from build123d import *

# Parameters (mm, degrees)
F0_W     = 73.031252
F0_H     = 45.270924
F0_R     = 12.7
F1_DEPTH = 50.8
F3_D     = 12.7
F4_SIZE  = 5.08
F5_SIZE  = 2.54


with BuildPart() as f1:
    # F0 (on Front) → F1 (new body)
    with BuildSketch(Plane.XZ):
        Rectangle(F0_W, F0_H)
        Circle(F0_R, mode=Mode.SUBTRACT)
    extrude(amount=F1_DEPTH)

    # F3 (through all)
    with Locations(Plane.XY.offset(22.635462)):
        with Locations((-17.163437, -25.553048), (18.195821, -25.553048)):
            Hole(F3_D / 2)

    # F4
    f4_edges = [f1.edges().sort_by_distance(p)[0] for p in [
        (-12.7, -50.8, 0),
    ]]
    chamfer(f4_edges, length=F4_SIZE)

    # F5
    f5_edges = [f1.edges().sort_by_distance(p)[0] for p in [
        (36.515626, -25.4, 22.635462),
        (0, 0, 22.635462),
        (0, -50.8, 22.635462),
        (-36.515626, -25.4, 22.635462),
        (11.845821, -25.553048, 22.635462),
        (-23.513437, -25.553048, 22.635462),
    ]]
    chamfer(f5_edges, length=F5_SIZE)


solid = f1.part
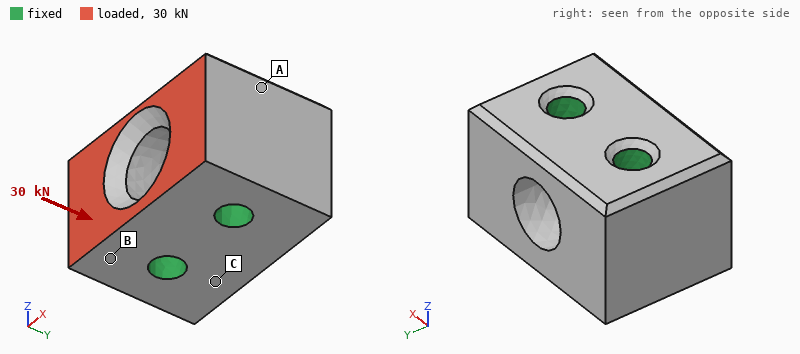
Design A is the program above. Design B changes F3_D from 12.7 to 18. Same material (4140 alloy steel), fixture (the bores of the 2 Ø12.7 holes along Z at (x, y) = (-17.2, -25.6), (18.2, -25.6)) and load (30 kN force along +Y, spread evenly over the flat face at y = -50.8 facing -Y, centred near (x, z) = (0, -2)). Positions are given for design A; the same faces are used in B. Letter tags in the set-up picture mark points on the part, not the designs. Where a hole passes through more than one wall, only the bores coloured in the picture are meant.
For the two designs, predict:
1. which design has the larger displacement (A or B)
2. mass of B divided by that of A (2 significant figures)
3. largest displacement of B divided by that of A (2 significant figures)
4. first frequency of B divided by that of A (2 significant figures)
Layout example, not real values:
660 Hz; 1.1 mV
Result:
A; 0.92; 0.83; 1.3
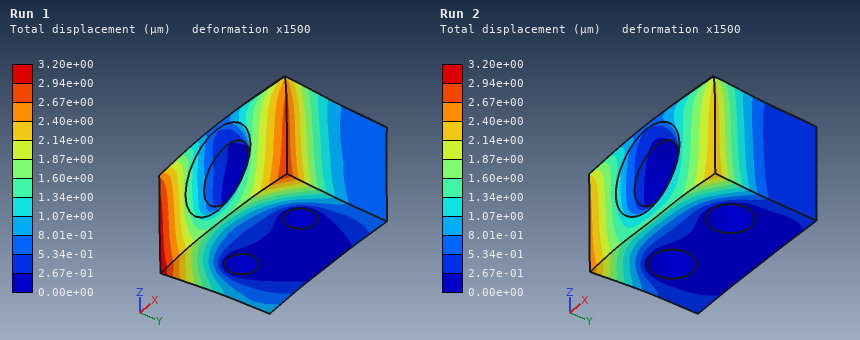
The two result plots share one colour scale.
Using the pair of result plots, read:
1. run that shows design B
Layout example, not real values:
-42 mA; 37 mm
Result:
Run 2
